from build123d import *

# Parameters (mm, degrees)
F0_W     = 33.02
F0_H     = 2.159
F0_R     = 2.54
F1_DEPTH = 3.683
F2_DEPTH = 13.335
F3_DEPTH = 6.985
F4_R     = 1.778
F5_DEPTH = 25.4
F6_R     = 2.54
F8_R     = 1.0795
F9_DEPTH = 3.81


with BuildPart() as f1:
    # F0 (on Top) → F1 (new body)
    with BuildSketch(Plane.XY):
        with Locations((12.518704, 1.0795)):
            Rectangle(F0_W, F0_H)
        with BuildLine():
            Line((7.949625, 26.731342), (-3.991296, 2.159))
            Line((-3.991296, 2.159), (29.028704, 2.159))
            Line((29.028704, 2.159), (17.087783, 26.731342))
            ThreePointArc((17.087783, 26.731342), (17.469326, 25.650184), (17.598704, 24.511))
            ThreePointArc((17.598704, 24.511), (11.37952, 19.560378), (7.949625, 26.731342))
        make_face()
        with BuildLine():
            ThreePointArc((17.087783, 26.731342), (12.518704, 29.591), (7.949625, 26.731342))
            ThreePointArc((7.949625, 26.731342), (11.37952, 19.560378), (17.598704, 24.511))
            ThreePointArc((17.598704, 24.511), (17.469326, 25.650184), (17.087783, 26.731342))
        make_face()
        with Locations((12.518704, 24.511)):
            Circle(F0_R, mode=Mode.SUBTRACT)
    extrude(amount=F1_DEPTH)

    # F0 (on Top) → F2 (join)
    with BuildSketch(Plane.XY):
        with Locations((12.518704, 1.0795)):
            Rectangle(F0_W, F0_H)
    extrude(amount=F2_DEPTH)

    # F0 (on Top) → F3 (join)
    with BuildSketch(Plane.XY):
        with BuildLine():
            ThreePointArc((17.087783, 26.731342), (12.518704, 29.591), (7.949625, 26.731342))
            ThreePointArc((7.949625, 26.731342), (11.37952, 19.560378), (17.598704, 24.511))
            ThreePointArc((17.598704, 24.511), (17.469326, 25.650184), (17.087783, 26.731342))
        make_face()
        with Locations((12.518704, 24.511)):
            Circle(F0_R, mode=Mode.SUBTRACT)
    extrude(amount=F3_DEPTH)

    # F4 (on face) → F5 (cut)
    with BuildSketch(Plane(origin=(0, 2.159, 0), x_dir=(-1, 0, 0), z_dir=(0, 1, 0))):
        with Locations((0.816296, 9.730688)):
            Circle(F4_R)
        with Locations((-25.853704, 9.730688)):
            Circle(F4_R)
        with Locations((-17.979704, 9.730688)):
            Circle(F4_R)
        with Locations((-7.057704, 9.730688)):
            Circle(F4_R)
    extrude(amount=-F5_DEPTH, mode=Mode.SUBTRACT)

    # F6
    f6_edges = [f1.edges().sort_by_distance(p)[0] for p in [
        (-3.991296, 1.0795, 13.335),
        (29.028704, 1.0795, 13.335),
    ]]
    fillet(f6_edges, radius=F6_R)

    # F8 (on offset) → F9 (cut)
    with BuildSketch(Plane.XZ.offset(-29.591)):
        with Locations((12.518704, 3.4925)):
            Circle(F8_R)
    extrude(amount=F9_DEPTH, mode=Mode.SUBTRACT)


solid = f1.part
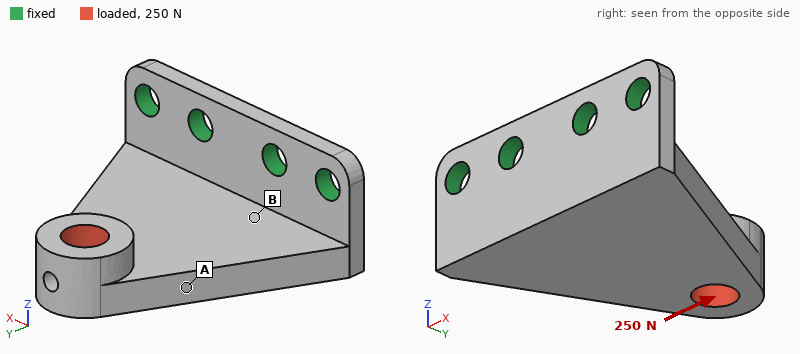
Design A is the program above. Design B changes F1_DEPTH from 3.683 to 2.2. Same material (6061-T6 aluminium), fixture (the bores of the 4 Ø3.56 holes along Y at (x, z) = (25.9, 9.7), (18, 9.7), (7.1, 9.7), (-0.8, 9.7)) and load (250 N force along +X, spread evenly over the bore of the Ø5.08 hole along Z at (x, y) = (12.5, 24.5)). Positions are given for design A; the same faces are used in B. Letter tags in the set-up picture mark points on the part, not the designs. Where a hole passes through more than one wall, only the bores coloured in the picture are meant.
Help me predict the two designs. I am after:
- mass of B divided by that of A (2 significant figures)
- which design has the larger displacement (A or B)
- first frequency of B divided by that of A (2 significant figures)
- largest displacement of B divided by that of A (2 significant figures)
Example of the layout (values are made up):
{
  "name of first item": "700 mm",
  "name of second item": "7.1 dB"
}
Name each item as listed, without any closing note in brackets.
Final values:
{
  "mass of B divided by that of A": "0.77",
  "which design has the larger displacement": "B",
  "first frequency of B divided by that of A": "0.80",
  "largest displacement of B divided by that of A": "2.5"
}
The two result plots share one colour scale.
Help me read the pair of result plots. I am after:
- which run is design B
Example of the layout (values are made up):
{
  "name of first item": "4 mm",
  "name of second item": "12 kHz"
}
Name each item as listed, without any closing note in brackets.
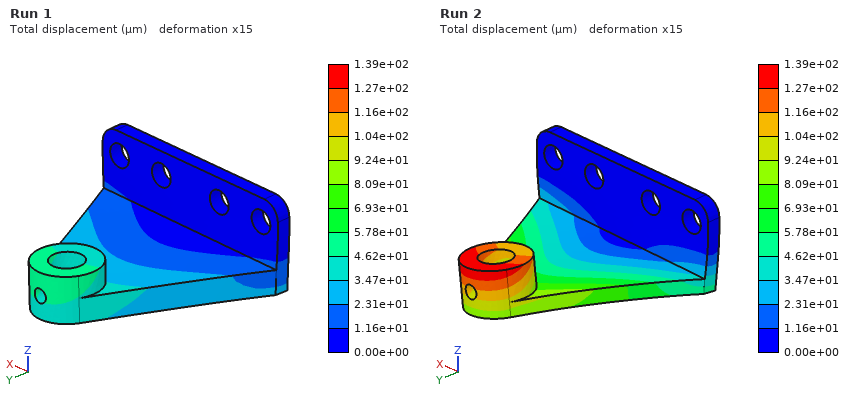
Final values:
{
  "which run is design B": "Run 2"
}
